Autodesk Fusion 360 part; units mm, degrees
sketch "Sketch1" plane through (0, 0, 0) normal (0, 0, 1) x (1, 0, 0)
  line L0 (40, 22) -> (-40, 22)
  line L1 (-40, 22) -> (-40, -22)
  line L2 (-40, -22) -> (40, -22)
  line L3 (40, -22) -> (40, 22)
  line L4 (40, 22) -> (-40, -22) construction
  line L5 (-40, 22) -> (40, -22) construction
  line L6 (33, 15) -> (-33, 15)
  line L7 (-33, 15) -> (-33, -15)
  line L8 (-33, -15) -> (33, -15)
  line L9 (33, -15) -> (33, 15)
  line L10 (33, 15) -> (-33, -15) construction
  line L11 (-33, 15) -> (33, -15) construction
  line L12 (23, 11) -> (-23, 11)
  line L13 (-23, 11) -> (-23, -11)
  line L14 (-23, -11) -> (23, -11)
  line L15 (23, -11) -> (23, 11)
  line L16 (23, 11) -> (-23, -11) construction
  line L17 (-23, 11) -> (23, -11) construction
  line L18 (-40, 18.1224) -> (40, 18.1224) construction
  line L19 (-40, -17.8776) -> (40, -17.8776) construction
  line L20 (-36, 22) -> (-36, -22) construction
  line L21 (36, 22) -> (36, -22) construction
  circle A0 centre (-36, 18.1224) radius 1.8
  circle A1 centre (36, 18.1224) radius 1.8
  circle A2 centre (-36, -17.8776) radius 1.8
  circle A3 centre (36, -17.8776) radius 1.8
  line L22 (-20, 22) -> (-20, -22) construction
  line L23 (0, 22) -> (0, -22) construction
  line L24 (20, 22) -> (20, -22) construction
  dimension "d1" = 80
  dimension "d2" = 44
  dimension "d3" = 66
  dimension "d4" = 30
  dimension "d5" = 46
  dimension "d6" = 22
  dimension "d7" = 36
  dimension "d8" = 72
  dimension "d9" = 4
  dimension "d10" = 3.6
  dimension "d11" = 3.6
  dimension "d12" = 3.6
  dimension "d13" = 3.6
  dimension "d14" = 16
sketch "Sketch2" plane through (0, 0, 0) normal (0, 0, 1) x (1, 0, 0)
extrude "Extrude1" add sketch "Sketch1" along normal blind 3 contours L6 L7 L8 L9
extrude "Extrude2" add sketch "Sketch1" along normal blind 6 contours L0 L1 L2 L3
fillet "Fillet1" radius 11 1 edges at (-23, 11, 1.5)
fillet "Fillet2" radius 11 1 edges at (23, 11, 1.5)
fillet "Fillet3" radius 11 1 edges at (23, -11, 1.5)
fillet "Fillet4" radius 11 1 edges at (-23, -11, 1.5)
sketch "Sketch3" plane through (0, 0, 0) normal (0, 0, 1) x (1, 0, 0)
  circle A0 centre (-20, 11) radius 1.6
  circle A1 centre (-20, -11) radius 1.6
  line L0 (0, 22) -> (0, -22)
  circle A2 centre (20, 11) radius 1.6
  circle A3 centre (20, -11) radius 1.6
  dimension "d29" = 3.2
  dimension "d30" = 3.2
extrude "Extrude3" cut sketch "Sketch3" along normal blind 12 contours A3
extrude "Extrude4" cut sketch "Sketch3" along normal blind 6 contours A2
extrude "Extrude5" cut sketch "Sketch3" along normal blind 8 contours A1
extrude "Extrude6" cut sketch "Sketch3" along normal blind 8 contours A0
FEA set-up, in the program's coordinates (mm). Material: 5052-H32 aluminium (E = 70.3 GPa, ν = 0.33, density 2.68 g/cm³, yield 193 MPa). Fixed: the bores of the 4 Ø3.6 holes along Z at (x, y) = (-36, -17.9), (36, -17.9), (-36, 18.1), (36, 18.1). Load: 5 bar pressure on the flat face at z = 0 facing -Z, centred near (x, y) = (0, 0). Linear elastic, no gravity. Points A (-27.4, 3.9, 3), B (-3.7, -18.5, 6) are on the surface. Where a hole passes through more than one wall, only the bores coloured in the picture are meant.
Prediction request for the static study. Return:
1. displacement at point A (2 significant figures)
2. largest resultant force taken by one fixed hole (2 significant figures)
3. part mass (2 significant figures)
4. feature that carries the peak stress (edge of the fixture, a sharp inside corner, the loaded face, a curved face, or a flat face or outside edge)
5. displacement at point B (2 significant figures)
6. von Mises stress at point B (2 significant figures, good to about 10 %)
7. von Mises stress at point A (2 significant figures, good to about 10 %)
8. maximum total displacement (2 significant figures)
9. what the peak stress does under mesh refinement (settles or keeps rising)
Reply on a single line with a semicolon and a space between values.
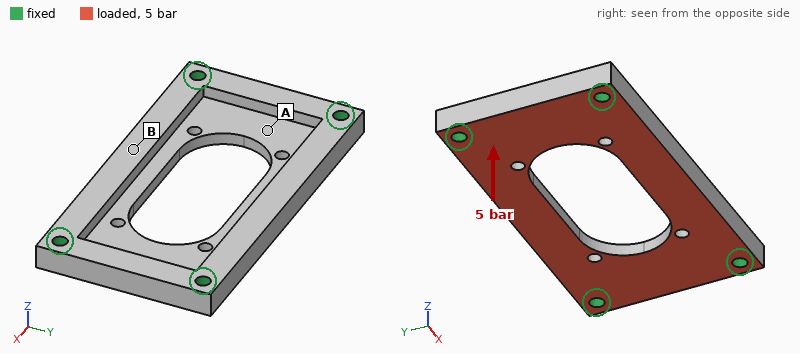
13 µm; 320 N; 32 g; edge of the fixture; 37 µm; 24 MPa; 8.1 MPa; 45 µm; keeps rising
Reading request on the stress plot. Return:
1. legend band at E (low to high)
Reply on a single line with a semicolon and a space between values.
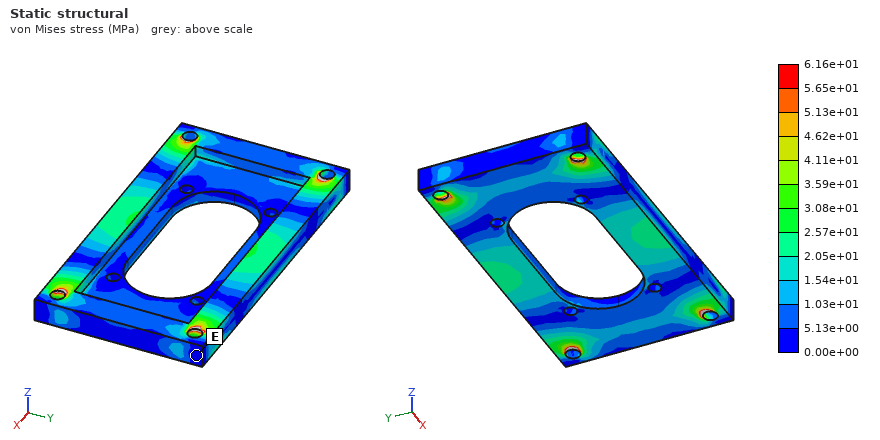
0.00e+00 to 5.13e+00 MPa
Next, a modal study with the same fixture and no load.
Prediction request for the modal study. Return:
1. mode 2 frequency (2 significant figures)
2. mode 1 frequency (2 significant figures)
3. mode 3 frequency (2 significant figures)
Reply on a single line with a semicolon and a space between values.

6100 Hz; 5900 Hz; 12 kHz
